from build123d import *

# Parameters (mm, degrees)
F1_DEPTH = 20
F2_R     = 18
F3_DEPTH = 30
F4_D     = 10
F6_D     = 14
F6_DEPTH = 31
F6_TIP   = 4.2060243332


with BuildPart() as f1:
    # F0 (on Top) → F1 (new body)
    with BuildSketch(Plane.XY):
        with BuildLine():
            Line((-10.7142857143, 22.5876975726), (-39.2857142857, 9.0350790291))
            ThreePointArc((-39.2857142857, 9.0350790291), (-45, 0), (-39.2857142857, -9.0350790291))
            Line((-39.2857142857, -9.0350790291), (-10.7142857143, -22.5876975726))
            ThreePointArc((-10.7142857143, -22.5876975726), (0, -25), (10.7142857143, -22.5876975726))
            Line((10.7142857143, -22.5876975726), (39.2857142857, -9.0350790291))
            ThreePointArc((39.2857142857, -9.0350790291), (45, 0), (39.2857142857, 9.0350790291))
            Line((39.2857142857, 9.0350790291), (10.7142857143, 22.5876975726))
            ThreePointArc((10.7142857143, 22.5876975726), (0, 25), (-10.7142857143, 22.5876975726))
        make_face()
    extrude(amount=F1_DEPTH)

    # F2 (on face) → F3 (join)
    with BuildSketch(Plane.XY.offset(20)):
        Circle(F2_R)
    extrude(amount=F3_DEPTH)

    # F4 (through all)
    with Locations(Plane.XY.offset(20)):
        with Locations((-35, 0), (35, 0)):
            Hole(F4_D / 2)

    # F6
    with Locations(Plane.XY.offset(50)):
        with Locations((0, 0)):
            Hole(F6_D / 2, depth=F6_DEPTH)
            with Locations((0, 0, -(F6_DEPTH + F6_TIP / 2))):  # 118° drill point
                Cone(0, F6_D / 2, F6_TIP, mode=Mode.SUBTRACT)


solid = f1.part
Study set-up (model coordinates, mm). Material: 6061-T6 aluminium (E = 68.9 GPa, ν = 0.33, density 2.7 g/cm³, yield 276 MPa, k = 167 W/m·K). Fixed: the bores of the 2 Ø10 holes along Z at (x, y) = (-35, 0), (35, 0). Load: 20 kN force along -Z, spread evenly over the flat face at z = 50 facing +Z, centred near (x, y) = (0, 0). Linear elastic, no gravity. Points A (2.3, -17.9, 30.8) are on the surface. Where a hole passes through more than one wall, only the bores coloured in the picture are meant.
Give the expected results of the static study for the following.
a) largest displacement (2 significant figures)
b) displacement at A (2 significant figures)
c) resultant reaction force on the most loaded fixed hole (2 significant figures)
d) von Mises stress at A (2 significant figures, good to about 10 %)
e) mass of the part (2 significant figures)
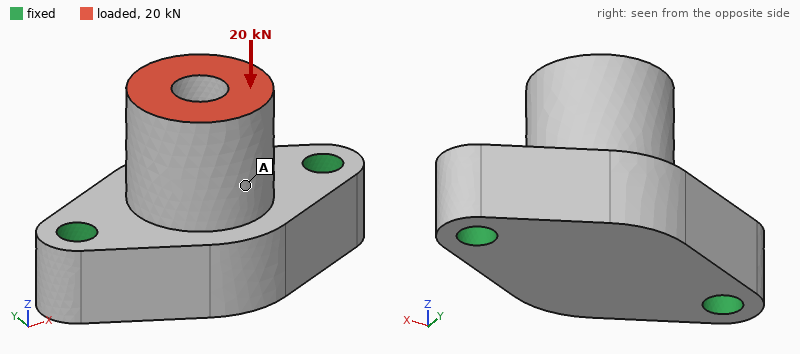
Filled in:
35 µm
29 µm
10 kN
15 MPa
220 g
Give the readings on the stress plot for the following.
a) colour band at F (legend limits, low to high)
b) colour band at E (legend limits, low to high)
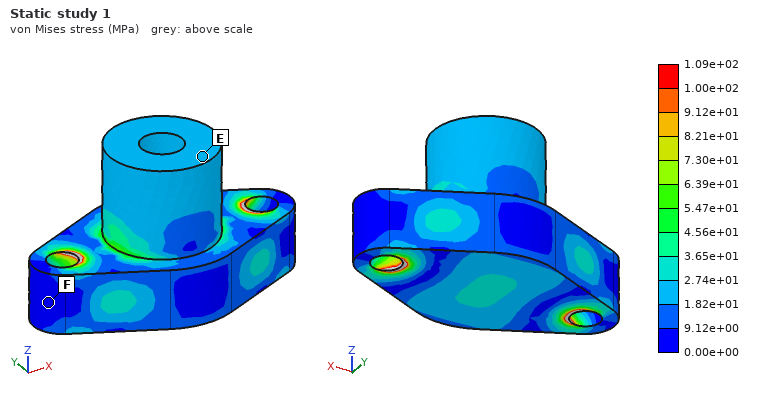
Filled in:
0.00e+00 to 9.12e+00 MPa
1.82e+01 to 2.74e+01 MPa
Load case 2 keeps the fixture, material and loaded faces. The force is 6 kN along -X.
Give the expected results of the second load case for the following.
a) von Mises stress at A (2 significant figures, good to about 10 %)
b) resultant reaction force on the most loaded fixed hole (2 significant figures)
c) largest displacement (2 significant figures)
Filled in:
15 MPa
5.2 kN
45 µm
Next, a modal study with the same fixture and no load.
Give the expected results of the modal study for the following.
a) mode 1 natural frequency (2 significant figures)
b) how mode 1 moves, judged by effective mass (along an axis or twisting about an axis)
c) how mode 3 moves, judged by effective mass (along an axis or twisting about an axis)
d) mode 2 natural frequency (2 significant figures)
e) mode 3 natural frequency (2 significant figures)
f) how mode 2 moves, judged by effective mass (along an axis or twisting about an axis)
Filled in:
6000 Hz
along Y
along X
11 kHz
11 kHz
along Z
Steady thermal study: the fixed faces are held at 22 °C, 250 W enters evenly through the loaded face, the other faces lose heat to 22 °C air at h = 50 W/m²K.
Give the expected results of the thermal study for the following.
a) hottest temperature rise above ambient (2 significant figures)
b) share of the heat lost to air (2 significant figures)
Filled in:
81 K
7.9 %
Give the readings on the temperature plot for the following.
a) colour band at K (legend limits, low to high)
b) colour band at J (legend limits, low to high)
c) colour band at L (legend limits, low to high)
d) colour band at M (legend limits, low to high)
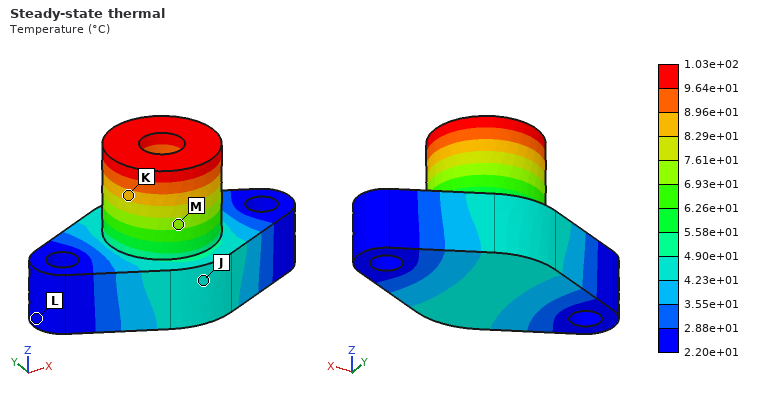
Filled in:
8.29e+01 to 8.96e+01 °C
4.23e+01 to 4.90e+01 °C
2.20e+01 to 2.88e+01 °C
6.93e+01 to 7.61e+01 °C
